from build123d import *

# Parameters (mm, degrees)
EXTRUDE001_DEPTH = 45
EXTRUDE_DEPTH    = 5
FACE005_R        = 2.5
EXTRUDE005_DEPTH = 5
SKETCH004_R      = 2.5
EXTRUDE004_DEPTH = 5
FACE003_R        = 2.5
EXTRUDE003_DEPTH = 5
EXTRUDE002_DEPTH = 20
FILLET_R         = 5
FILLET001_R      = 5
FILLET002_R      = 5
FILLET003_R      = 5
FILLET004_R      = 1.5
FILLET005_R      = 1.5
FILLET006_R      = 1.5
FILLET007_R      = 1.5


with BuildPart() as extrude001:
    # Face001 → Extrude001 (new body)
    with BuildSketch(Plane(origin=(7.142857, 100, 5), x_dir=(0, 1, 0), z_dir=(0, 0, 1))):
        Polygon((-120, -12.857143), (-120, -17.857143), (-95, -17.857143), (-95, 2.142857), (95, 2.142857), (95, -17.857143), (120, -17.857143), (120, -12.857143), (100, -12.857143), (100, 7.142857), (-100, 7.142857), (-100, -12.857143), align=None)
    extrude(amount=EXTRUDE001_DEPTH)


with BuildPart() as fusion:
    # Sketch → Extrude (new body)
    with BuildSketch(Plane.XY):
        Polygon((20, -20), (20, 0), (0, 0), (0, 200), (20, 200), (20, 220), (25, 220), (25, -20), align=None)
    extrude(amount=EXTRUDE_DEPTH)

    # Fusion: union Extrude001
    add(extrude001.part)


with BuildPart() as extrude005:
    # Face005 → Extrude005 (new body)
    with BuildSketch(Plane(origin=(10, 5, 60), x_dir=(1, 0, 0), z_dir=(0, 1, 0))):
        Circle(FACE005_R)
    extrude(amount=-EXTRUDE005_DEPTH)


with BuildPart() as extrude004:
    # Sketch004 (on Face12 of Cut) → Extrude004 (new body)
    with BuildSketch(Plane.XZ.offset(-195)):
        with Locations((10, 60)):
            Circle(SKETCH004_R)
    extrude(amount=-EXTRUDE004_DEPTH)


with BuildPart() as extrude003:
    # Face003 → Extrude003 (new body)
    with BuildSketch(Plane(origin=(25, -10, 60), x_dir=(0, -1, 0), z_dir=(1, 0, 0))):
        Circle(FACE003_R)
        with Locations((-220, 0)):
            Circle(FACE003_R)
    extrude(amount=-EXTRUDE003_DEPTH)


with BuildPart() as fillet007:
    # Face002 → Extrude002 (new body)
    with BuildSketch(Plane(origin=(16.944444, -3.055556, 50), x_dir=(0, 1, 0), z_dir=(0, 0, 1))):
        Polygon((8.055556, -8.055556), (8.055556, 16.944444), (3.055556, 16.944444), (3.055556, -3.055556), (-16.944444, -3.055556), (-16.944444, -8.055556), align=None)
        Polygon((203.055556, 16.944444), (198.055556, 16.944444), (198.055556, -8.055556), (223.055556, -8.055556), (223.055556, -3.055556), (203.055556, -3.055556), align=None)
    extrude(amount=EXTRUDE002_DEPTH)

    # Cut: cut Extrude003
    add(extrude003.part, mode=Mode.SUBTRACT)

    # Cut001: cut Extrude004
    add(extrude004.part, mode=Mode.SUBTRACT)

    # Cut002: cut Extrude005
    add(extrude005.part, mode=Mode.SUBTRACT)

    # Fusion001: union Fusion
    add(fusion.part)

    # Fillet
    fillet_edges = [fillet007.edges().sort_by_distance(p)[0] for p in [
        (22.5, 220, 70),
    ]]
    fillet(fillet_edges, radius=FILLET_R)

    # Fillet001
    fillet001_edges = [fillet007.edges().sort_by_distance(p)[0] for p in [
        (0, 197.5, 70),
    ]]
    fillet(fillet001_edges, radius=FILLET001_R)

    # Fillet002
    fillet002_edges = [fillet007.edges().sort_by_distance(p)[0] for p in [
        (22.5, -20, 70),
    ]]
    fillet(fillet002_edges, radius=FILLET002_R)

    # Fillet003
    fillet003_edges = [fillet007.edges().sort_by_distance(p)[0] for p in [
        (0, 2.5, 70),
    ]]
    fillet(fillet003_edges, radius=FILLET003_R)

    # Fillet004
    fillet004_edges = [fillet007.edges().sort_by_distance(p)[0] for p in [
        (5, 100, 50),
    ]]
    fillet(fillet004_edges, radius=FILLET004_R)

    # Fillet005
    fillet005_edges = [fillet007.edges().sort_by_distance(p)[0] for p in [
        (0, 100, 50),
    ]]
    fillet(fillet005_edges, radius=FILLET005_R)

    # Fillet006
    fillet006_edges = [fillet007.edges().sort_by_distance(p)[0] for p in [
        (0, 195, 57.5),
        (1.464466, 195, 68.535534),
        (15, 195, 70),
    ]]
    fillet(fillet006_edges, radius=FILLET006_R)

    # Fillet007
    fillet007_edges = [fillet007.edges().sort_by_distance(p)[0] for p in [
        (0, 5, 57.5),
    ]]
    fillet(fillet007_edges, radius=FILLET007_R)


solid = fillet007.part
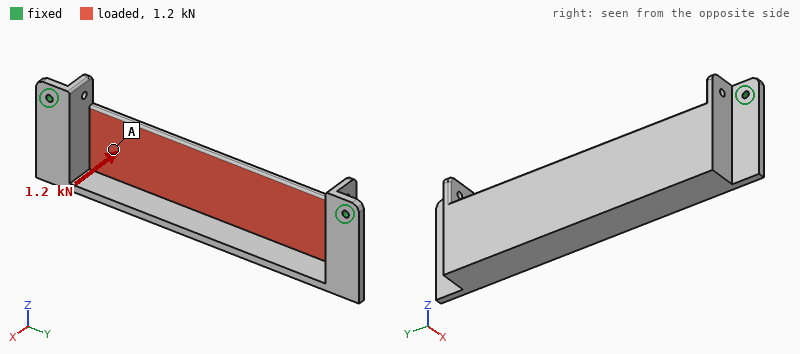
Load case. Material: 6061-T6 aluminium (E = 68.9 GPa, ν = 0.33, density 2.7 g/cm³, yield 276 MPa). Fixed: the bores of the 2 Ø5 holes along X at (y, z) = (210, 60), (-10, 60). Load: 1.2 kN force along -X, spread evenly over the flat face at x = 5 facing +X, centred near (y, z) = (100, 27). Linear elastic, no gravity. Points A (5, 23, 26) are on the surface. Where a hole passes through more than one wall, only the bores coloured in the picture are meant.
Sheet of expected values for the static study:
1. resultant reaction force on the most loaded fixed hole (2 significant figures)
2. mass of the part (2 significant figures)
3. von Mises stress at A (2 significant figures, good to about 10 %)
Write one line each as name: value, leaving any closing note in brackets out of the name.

resultant reaction force on the most loaded fixed hole: 790 N
mass of the part: 260 g
von Mises stress at A: 19 MPa
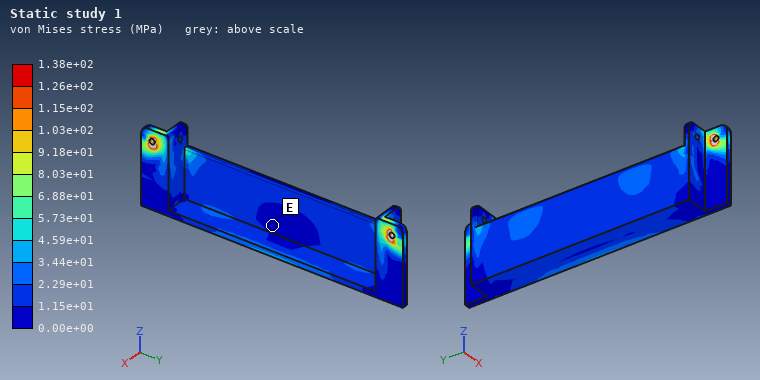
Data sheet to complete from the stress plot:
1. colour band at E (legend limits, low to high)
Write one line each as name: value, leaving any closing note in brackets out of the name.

colour band at E: 0.00e+00 to 1.15e+01 MPa
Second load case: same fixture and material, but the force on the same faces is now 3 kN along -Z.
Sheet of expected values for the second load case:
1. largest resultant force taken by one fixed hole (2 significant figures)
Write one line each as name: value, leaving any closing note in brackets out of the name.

largest resultant force taken by one fixed hole: 1.5 kN
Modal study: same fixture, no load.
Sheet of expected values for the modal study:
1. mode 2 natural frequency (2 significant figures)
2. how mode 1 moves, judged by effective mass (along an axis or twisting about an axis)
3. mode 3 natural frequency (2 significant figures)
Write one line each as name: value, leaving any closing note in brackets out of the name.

mode 2 natural frequency: 1000 Hz
how mode 1 moves, judged by effective mass: along X
mode 3 natural frequency: 1200 Hz
